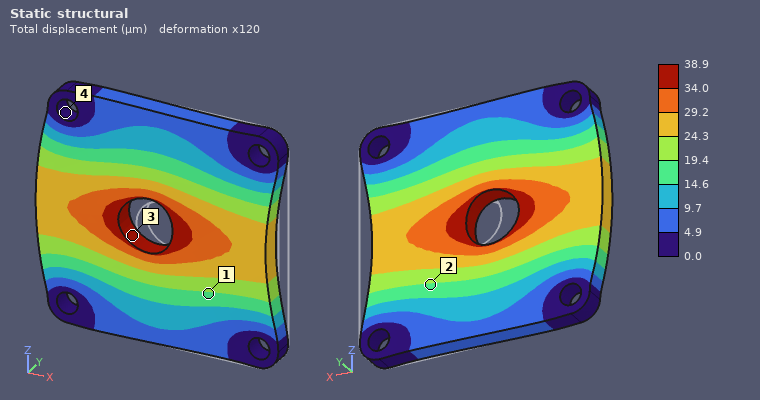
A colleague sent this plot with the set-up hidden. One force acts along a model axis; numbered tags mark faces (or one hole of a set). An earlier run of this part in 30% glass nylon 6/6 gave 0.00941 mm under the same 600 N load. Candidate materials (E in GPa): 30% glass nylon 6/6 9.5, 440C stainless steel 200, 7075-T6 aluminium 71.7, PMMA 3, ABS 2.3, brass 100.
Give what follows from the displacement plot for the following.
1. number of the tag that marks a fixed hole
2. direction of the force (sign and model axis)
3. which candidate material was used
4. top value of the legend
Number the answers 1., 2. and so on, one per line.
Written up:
1. 4
2. -X
3. ABS
4. 38.9 µm
